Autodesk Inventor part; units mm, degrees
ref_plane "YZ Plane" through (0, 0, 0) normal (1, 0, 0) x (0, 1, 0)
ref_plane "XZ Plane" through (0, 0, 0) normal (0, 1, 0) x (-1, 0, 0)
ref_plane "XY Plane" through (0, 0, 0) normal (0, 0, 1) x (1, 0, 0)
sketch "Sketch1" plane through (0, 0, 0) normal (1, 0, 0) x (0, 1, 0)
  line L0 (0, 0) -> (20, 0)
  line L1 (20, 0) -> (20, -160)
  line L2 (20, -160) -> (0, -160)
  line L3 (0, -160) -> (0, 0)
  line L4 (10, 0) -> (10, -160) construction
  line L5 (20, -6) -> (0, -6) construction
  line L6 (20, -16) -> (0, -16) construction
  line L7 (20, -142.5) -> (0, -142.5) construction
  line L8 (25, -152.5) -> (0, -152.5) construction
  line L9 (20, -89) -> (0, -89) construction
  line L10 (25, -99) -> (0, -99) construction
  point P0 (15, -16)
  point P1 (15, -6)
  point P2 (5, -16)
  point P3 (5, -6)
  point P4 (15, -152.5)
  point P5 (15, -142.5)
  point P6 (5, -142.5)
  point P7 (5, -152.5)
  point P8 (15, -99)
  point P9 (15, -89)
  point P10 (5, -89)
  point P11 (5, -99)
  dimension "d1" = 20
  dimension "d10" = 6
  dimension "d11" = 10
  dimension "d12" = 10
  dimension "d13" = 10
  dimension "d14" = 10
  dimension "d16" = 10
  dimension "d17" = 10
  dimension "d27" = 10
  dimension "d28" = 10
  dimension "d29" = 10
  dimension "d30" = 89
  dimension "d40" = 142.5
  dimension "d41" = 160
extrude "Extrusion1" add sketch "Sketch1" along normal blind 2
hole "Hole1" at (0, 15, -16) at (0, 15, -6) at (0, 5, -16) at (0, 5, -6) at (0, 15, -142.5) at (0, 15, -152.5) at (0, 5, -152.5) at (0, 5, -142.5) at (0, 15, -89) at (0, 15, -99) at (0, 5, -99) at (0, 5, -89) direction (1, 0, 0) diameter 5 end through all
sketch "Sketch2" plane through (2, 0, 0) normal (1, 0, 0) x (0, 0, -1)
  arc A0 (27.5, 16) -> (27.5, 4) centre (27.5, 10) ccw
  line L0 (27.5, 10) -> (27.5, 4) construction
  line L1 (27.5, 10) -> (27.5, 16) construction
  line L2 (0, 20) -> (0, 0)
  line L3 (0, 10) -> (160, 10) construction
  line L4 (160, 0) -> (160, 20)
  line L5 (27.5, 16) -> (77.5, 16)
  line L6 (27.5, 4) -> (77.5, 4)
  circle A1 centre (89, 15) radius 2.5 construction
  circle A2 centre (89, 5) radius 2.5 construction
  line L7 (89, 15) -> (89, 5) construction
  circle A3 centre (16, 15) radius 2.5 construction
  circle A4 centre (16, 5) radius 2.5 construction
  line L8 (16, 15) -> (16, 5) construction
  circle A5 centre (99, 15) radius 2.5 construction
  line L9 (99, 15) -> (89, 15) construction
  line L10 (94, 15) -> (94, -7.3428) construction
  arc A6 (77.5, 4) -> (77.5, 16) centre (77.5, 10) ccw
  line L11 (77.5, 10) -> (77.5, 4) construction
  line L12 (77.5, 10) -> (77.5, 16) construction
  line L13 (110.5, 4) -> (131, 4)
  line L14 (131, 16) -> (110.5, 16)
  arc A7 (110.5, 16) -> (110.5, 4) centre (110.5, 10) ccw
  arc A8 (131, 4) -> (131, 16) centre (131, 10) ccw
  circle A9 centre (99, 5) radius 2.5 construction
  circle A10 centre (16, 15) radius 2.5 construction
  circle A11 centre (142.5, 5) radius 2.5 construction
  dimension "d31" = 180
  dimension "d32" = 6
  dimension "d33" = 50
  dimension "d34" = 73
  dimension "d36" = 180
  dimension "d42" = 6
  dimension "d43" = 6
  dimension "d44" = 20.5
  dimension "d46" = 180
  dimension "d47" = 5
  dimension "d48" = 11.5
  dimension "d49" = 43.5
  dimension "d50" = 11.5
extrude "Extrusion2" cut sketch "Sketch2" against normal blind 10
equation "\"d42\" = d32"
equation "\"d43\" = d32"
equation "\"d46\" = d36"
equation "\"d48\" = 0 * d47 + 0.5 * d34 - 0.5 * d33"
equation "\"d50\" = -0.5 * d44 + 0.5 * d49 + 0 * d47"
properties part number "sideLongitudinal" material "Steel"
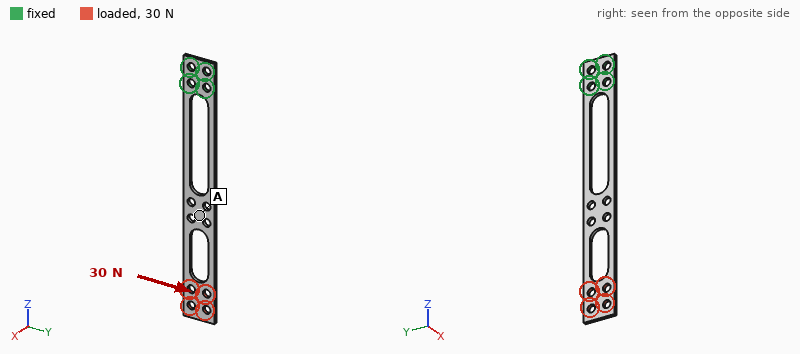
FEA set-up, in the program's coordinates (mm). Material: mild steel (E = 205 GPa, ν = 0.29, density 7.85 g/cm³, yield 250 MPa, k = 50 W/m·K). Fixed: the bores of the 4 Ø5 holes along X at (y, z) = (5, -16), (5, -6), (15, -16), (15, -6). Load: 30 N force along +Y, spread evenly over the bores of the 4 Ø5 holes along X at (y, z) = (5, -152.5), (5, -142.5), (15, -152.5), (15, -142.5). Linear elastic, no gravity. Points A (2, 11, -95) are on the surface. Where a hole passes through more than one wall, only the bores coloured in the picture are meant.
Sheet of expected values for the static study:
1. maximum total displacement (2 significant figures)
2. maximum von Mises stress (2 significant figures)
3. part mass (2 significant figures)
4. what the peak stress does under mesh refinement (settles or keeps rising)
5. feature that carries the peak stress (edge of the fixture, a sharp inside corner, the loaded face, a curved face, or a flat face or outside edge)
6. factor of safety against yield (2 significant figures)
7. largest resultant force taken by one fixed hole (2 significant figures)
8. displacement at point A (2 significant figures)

0.26 mm
95 MPa
30 g
settles
a flat face or outside edge
2.6
220 N
0.17 mm
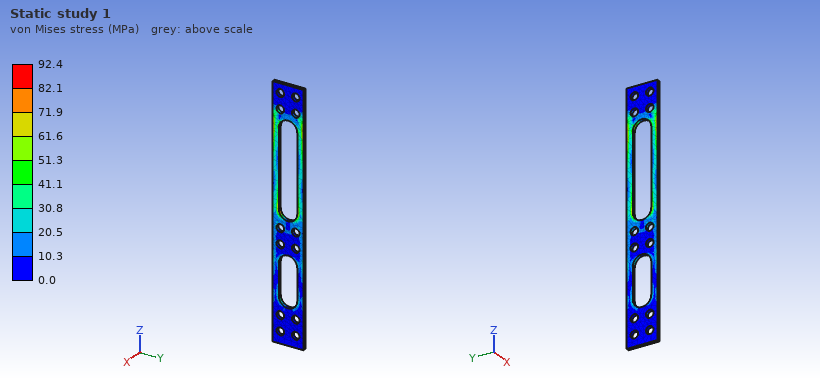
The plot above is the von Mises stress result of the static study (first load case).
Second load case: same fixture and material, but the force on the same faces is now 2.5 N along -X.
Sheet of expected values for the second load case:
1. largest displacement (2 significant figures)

1.7 mm
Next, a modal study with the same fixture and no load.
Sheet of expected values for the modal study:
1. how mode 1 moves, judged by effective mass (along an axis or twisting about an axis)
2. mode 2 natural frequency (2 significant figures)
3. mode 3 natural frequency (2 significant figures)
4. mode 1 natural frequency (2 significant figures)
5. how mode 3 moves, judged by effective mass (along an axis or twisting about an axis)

along X
450 Hz
480 Hz
66 Hz
along Y
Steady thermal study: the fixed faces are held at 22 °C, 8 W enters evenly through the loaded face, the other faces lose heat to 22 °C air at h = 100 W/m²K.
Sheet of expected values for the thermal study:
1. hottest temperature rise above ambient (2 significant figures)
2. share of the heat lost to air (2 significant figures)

67 K
100 %
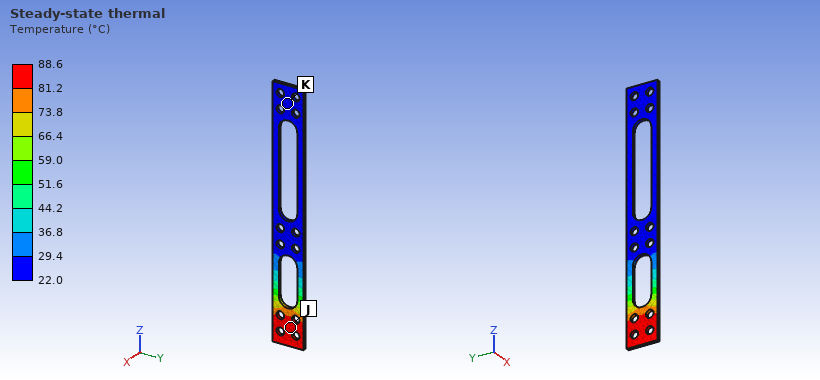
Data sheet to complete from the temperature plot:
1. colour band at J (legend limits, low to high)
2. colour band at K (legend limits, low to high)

81.2 to 88.6 °C
22.0 to 29.4 °C
